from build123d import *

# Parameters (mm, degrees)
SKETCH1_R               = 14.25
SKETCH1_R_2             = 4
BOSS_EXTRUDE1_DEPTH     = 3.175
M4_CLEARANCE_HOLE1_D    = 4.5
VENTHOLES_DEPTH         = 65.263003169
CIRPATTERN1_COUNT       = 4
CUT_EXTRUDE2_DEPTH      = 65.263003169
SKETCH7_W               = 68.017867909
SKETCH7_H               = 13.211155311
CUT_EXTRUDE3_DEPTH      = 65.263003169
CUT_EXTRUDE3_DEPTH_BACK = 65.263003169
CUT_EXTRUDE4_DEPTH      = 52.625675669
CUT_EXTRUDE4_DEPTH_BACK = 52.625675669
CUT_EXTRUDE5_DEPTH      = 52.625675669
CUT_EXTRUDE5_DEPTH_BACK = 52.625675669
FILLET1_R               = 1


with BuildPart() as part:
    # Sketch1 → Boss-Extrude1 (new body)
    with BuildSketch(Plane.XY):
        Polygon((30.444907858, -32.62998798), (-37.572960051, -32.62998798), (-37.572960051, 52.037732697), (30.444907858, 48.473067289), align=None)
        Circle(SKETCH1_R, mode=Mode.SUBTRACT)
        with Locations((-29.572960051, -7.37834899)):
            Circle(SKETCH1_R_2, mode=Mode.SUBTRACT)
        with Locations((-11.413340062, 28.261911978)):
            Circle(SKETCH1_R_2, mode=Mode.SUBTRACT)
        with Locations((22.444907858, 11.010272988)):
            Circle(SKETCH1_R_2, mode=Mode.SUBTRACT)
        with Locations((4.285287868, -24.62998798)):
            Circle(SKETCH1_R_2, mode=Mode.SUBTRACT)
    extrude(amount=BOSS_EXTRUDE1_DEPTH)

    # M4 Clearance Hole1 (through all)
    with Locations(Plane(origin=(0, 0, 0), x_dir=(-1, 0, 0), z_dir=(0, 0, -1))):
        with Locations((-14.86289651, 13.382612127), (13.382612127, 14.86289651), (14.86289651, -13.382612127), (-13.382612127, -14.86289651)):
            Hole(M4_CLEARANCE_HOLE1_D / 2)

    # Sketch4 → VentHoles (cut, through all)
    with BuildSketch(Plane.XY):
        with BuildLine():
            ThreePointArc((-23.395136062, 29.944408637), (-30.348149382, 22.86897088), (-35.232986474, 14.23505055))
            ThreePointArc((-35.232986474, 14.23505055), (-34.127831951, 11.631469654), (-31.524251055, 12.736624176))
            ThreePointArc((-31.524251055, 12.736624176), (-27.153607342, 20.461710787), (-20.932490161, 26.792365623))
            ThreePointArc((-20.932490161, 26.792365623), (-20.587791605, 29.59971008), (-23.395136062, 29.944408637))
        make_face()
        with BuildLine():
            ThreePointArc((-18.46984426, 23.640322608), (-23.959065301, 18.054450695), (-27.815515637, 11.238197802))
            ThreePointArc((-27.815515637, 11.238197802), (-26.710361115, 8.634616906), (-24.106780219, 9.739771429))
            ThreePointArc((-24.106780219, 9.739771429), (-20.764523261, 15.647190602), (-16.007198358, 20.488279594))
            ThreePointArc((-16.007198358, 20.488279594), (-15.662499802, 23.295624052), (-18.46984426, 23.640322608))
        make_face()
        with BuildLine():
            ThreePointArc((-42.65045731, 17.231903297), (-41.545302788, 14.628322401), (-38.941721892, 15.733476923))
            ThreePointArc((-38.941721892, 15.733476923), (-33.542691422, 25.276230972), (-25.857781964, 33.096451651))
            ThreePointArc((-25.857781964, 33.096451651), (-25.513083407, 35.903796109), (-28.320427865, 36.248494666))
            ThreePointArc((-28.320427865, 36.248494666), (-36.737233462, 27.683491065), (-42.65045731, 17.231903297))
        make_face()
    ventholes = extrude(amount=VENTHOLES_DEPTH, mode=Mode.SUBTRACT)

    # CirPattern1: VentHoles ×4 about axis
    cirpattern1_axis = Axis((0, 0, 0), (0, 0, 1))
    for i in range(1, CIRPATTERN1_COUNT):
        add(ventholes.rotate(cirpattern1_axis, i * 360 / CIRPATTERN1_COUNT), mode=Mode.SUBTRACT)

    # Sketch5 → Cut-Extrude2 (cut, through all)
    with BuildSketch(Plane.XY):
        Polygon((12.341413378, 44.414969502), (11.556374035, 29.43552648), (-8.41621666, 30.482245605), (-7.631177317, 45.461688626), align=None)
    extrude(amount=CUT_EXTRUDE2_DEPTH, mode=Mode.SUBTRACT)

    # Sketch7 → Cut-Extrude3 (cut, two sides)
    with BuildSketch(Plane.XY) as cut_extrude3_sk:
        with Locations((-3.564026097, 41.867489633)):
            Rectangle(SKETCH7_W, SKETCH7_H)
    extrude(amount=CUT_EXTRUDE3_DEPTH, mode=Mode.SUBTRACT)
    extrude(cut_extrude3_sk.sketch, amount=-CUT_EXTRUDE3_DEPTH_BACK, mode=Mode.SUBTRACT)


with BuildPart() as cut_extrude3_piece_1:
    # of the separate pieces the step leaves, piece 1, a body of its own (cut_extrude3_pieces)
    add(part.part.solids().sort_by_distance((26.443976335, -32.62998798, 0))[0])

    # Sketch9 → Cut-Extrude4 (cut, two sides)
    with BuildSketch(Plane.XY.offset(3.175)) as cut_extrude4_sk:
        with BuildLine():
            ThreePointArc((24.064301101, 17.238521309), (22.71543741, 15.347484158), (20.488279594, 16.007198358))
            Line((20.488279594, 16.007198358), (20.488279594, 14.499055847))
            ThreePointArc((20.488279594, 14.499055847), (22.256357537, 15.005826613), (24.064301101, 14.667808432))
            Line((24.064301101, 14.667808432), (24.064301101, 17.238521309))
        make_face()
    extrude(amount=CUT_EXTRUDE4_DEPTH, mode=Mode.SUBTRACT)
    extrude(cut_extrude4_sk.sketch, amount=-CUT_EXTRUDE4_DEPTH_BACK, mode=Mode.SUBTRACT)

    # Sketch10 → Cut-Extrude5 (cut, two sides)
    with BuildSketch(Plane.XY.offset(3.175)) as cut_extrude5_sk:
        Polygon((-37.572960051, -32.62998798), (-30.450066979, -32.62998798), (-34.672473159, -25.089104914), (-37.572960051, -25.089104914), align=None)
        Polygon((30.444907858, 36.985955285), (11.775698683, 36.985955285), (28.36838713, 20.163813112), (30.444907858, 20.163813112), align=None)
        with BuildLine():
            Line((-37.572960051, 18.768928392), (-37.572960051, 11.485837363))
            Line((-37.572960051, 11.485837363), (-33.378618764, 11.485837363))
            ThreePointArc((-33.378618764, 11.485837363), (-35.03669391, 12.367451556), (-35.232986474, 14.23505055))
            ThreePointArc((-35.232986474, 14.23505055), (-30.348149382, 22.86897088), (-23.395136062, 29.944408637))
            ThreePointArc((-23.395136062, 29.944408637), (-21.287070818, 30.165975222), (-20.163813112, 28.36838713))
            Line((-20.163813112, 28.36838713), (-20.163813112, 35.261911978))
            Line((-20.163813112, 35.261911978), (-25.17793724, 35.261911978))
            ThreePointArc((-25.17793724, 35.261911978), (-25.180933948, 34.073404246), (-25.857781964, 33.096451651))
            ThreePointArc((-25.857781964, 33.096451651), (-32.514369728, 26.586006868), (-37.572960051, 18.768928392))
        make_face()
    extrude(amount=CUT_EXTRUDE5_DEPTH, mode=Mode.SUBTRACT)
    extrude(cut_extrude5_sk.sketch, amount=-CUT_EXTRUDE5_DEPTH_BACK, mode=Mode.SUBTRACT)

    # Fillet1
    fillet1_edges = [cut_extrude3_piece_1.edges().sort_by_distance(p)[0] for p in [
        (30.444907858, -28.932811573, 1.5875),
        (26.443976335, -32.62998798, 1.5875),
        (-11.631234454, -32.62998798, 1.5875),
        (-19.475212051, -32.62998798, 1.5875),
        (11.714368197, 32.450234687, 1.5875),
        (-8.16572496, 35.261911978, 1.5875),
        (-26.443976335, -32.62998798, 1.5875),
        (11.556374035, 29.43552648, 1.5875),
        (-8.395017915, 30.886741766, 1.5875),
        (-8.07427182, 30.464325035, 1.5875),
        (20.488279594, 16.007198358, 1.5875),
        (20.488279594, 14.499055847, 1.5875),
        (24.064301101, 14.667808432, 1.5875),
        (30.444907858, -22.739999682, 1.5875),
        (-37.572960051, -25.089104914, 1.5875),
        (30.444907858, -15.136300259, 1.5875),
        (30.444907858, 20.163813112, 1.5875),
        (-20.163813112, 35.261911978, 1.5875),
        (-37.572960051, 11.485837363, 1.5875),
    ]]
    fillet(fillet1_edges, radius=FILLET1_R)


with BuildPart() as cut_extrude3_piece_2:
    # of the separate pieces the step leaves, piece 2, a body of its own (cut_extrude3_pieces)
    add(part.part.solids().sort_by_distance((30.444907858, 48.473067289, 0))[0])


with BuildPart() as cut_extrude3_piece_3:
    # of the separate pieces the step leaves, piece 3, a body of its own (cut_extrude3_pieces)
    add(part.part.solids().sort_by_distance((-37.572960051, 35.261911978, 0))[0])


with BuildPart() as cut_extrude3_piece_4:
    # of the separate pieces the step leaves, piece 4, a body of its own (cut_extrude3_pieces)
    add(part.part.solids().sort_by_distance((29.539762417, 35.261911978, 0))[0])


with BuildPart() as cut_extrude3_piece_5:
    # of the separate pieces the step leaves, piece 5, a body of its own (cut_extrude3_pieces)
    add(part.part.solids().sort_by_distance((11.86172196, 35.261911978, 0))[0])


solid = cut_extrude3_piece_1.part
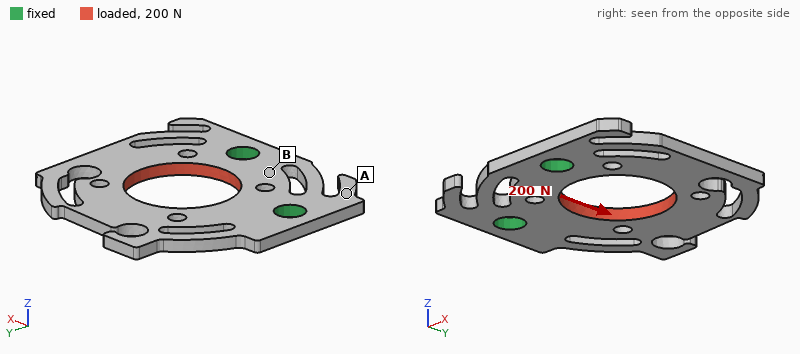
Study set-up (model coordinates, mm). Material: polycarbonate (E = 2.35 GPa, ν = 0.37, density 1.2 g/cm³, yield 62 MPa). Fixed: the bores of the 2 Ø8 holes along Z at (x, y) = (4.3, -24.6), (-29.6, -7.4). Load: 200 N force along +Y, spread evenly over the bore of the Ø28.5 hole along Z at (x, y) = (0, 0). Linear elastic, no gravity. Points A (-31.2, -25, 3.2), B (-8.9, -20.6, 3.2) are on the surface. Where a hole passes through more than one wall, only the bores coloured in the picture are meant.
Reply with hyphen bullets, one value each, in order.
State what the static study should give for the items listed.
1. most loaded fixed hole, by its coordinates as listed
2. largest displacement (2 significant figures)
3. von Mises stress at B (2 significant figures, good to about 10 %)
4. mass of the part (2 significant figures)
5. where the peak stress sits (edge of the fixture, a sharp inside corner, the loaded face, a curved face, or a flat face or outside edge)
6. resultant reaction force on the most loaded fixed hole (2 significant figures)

- (4.3, -24.6)
- 0.12 mm
- 1.6 MPa
- 10 g
- a curved face
- 140 N
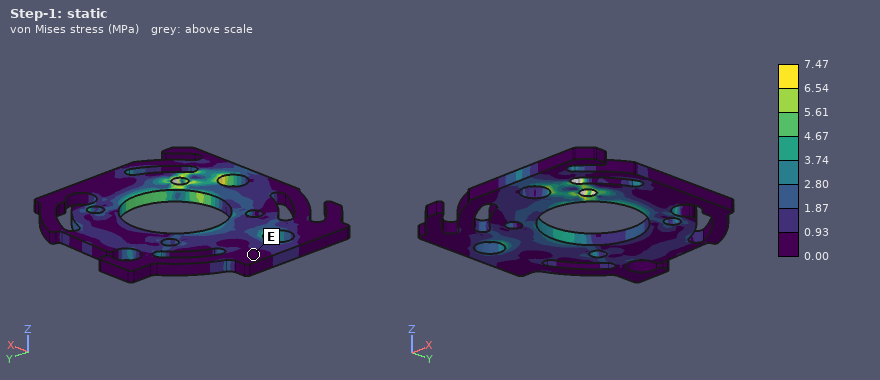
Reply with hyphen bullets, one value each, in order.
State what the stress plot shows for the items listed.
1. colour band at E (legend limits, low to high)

- 0.00 to 0.93 MPa
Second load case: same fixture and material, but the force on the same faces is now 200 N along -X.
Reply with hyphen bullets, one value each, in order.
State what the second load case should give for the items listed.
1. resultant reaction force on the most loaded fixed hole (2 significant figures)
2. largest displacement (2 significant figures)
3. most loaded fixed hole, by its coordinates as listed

- 120 N
- 0.16 mm
- (-29.6, -7.4)
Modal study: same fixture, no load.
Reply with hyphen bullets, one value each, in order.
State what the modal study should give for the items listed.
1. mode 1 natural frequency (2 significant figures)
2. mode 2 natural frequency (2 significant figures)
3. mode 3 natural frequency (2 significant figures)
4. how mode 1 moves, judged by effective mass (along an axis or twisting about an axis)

- 300 Hz
- 660 Hz
- 1300 Hz
- along Z
